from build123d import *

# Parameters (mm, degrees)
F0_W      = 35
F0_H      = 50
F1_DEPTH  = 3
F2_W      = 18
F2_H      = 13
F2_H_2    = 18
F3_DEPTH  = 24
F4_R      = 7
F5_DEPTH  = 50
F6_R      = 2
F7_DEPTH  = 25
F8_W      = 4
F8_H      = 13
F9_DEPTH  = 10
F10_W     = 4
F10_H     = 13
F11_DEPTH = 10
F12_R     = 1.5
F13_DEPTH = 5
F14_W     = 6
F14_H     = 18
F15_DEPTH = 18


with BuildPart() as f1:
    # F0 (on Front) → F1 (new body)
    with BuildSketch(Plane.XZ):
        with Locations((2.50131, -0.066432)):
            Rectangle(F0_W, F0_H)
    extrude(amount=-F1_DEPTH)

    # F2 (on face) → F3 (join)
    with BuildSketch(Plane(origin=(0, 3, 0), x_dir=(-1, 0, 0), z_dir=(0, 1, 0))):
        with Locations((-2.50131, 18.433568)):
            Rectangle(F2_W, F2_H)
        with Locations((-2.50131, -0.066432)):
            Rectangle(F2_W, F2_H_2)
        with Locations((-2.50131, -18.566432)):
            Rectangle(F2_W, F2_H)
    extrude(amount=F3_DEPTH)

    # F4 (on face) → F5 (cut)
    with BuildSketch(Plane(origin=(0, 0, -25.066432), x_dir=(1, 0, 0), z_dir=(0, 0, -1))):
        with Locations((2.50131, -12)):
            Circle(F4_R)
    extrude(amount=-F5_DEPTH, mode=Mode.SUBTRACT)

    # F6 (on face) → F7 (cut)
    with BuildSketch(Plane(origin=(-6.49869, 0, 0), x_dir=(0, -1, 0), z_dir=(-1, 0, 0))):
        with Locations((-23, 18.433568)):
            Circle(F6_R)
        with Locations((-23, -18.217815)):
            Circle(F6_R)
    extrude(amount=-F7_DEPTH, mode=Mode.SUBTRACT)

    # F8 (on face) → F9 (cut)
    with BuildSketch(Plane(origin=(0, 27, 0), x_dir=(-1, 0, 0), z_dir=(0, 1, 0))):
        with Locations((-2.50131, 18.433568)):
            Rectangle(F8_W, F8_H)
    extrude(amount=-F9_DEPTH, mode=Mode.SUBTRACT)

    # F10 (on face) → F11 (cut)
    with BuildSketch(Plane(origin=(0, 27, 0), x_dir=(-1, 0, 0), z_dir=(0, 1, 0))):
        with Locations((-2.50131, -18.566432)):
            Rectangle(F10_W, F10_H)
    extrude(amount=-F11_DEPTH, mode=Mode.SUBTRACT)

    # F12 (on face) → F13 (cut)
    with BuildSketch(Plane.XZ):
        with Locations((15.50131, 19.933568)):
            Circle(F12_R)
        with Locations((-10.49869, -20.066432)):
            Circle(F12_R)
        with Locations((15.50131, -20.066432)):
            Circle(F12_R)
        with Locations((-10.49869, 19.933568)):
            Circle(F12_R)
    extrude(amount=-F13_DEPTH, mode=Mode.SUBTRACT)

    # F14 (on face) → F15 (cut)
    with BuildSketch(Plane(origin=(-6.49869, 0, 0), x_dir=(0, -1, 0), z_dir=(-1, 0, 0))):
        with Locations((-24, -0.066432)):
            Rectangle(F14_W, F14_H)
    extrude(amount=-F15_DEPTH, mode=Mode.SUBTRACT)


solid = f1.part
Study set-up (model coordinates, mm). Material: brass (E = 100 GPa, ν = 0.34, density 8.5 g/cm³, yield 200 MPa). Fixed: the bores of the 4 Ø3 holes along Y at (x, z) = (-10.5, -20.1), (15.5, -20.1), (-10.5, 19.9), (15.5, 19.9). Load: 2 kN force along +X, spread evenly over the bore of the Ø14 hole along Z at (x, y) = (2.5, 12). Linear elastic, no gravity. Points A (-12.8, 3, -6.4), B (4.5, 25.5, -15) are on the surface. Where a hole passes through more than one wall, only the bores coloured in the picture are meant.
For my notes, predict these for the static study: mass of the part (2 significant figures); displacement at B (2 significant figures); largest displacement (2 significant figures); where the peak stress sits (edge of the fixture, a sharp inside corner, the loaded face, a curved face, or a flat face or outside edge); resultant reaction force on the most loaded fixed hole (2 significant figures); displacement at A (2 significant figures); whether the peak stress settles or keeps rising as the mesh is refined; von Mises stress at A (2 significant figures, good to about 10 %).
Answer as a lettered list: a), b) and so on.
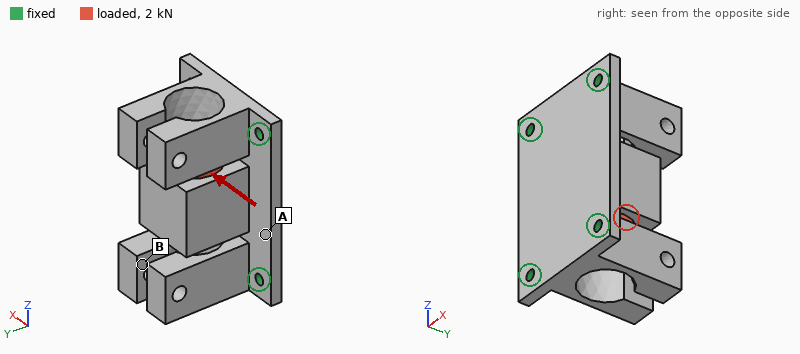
a) 120 g
b) 19 µm
c) 83 µm
d) edge of the fixture
e) 770 N
f) 29 µm
g) keeps rising
h) 40 MPa
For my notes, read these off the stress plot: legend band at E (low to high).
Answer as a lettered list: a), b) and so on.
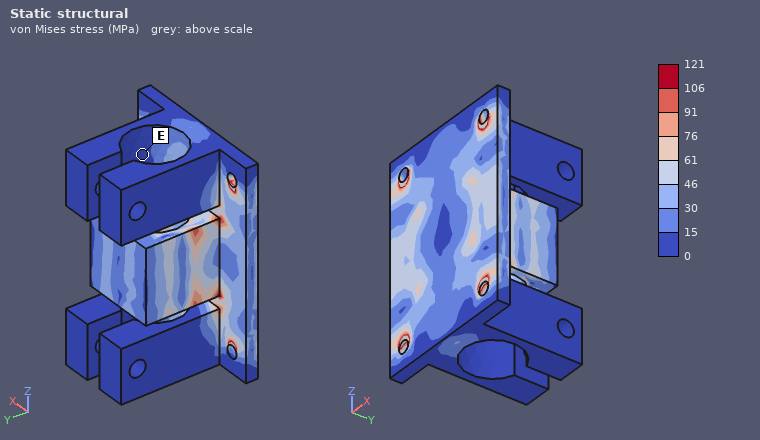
a) 0 to 15 MPa
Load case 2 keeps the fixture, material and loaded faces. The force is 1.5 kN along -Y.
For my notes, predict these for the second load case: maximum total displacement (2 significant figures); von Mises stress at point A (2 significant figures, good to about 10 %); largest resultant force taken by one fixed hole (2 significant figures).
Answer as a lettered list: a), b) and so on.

a) 52 µm
b) 34 MPa
c) 430 N
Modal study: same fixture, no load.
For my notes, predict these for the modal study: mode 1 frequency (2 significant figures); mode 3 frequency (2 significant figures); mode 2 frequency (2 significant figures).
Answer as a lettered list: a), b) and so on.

a) 1900 Hz
b) 2000 Hz
c) 2000 Hz
